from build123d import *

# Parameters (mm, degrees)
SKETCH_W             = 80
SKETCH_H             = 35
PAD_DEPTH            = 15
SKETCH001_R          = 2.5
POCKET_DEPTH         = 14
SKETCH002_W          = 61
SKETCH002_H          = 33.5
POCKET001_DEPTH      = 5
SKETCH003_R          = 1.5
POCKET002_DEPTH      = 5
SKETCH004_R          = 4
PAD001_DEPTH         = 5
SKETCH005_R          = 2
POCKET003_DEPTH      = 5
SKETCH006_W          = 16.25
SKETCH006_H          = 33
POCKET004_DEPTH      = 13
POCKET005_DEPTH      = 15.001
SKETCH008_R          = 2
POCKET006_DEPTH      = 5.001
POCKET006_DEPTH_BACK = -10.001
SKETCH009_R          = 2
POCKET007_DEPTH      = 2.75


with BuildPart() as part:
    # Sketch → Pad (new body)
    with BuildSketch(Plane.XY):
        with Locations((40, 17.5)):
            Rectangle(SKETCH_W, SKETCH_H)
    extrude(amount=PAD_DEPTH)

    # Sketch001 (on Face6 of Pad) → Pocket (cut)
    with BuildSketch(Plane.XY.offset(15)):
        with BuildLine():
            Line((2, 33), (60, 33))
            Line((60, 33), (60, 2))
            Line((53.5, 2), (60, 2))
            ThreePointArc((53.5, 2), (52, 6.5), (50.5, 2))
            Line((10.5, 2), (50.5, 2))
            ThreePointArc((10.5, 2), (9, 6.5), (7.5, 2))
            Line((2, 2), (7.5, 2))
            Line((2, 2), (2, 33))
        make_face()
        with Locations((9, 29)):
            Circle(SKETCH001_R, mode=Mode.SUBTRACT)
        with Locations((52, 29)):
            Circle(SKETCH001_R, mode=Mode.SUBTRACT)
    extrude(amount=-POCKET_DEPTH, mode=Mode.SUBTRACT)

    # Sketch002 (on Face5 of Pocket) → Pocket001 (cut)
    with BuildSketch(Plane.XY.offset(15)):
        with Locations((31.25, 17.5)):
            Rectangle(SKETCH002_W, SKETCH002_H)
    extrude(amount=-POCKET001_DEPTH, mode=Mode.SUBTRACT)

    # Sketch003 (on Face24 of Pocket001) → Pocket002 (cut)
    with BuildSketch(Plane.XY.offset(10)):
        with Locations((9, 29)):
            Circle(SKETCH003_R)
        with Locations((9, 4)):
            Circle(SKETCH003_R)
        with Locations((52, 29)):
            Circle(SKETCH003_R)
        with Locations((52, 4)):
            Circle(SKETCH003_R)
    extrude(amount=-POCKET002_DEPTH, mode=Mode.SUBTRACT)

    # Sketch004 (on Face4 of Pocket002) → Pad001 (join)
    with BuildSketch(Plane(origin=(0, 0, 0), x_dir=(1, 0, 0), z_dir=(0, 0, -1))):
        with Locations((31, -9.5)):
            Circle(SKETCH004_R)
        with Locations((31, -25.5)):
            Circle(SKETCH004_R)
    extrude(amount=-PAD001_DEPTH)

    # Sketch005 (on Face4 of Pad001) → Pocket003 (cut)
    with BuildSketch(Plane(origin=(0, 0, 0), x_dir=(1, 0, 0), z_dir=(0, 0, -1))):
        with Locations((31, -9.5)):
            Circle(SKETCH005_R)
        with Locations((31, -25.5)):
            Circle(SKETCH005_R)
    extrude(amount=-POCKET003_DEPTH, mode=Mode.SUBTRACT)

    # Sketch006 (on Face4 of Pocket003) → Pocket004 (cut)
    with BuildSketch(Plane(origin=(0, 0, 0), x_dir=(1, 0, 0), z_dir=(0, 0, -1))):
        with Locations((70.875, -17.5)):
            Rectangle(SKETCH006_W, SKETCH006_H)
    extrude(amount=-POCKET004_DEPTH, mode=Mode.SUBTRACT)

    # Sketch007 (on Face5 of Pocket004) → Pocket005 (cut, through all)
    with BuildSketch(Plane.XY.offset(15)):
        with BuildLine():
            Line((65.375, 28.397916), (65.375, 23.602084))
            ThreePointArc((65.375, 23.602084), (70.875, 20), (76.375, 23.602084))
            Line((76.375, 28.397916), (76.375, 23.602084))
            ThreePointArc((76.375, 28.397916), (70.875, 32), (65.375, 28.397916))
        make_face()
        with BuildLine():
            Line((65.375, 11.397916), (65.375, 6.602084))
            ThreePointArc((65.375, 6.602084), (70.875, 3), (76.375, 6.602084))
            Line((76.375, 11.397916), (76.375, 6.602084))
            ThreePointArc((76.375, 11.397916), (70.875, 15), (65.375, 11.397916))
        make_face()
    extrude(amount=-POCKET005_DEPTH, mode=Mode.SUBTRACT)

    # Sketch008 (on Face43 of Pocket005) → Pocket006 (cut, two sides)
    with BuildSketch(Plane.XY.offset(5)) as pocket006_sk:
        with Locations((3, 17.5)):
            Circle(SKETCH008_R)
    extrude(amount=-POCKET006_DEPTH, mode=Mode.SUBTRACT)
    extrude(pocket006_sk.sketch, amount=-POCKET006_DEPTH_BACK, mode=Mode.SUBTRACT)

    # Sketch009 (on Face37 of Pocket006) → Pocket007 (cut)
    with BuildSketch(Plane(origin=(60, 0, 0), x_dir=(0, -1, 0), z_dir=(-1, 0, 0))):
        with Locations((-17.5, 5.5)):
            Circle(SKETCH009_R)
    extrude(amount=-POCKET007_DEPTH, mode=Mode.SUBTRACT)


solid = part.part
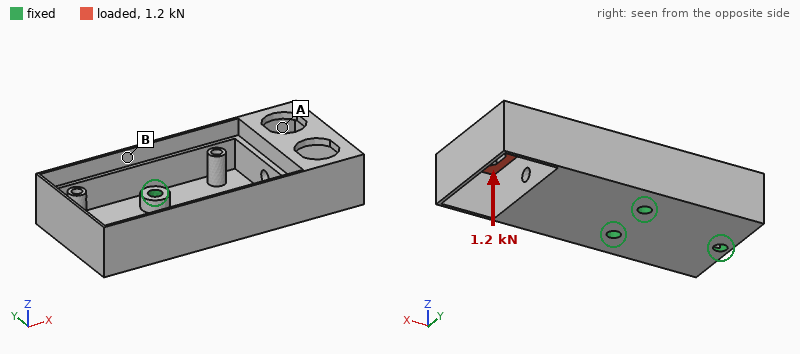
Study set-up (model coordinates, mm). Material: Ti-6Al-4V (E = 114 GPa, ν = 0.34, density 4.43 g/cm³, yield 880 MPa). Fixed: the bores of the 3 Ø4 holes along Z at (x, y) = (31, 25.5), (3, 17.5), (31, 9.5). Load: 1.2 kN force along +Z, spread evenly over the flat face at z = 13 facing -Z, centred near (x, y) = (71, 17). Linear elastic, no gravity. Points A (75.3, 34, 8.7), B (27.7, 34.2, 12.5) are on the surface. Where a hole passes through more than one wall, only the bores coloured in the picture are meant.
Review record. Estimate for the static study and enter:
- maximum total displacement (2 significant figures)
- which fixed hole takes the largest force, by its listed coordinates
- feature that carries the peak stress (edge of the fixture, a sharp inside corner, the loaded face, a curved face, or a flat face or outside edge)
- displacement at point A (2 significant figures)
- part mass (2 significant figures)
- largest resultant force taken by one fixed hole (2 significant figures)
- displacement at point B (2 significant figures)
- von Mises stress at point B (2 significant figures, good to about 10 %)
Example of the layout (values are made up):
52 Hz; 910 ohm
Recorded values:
1.0 mm; (3, 17.5); a flat face or outside edge; 0.90 mm; 40 g; 1.5 kN; 0.32 mm; 240 MPa
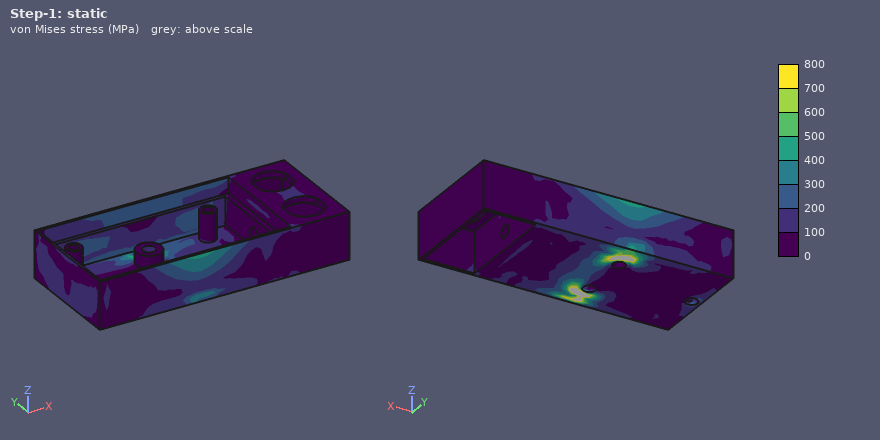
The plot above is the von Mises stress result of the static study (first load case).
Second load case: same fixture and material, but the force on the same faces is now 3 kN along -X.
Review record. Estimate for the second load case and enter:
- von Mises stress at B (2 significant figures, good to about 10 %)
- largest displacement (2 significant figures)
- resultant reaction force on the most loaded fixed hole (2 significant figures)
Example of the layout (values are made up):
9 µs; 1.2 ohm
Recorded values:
190 MPa; 0.65 mm; 1.4 kN
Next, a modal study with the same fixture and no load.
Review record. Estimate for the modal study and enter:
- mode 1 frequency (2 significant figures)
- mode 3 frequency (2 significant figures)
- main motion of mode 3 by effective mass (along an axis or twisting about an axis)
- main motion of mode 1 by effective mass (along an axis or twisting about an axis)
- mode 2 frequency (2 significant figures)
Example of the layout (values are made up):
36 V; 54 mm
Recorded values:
1600 Hz; 5100 Hz; along Y; along Z; 1800 Hz
